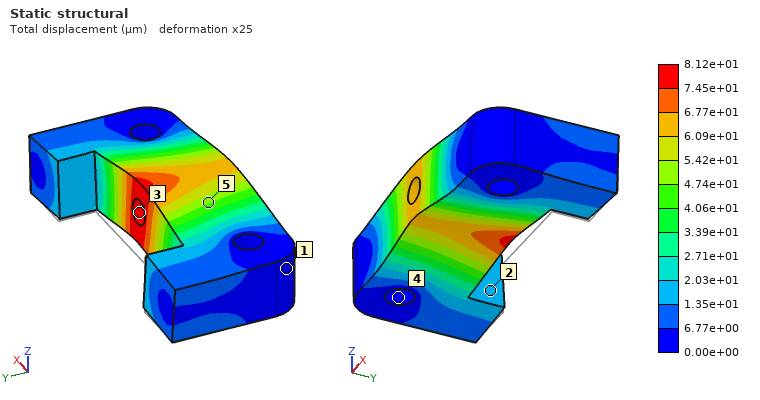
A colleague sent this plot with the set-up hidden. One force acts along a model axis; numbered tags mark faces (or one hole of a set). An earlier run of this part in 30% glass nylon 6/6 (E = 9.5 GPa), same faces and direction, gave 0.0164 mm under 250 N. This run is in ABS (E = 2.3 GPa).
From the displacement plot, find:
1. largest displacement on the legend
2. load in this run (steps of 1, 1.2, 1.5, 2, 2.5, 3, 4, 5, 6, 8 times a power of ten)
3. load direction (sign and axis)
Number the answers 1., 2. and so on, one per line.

1. 8.12e+01 µm
2. 300 N
3. +Z
